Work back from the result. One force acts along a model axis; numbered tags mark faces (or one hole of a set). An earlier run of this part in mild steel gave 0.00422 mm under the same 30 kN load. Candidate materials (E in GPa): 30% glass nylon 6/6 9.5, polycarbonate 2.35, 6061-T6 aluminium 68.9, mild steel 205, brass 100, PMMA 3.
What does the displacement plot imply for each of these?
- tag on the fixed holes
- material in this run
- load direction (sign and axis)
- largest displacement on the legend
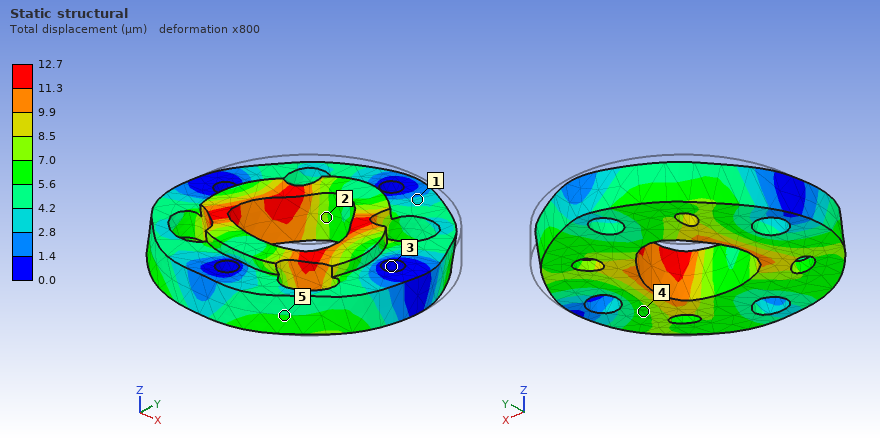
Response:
3
6061-T6 aluminium
-Y
12.7 µm
